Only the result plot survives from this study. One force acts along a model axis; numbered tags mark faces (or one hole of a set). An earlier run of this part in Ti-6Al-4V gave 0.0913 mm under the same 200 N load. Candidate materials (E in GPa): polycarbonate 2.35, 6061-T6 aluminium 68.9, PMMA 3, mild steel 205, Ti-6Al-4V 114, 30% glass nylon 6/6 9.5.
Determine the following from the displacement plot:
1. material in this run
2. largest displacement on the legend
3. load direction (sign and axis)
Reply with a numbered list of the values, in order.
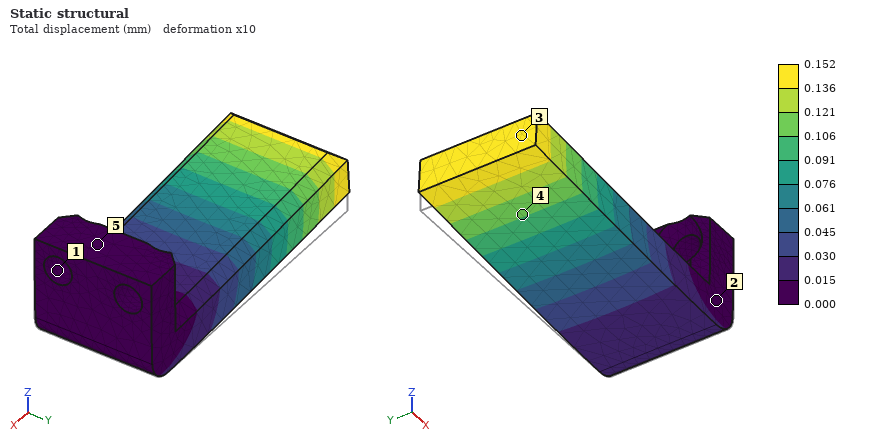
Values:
1. 6061-T6 aluminium
2. 0.152 mm
3. +Z
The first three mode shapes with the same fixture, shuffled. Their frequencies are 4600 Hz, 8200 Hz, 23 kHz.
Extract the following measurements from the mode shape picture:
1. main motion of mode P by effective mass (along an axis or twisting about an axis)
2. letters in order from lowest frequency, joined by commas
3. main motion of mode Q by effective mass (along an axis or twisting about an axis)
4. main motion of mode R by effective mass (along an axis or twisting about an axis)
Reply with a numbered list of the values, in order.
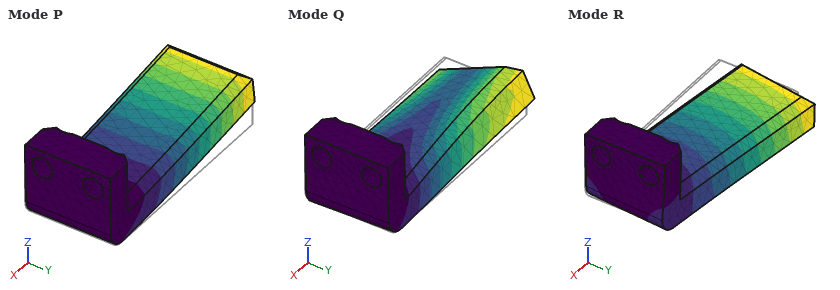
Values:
1. along Z
2. P, R, Q
3. twisting about X
4. along Y
